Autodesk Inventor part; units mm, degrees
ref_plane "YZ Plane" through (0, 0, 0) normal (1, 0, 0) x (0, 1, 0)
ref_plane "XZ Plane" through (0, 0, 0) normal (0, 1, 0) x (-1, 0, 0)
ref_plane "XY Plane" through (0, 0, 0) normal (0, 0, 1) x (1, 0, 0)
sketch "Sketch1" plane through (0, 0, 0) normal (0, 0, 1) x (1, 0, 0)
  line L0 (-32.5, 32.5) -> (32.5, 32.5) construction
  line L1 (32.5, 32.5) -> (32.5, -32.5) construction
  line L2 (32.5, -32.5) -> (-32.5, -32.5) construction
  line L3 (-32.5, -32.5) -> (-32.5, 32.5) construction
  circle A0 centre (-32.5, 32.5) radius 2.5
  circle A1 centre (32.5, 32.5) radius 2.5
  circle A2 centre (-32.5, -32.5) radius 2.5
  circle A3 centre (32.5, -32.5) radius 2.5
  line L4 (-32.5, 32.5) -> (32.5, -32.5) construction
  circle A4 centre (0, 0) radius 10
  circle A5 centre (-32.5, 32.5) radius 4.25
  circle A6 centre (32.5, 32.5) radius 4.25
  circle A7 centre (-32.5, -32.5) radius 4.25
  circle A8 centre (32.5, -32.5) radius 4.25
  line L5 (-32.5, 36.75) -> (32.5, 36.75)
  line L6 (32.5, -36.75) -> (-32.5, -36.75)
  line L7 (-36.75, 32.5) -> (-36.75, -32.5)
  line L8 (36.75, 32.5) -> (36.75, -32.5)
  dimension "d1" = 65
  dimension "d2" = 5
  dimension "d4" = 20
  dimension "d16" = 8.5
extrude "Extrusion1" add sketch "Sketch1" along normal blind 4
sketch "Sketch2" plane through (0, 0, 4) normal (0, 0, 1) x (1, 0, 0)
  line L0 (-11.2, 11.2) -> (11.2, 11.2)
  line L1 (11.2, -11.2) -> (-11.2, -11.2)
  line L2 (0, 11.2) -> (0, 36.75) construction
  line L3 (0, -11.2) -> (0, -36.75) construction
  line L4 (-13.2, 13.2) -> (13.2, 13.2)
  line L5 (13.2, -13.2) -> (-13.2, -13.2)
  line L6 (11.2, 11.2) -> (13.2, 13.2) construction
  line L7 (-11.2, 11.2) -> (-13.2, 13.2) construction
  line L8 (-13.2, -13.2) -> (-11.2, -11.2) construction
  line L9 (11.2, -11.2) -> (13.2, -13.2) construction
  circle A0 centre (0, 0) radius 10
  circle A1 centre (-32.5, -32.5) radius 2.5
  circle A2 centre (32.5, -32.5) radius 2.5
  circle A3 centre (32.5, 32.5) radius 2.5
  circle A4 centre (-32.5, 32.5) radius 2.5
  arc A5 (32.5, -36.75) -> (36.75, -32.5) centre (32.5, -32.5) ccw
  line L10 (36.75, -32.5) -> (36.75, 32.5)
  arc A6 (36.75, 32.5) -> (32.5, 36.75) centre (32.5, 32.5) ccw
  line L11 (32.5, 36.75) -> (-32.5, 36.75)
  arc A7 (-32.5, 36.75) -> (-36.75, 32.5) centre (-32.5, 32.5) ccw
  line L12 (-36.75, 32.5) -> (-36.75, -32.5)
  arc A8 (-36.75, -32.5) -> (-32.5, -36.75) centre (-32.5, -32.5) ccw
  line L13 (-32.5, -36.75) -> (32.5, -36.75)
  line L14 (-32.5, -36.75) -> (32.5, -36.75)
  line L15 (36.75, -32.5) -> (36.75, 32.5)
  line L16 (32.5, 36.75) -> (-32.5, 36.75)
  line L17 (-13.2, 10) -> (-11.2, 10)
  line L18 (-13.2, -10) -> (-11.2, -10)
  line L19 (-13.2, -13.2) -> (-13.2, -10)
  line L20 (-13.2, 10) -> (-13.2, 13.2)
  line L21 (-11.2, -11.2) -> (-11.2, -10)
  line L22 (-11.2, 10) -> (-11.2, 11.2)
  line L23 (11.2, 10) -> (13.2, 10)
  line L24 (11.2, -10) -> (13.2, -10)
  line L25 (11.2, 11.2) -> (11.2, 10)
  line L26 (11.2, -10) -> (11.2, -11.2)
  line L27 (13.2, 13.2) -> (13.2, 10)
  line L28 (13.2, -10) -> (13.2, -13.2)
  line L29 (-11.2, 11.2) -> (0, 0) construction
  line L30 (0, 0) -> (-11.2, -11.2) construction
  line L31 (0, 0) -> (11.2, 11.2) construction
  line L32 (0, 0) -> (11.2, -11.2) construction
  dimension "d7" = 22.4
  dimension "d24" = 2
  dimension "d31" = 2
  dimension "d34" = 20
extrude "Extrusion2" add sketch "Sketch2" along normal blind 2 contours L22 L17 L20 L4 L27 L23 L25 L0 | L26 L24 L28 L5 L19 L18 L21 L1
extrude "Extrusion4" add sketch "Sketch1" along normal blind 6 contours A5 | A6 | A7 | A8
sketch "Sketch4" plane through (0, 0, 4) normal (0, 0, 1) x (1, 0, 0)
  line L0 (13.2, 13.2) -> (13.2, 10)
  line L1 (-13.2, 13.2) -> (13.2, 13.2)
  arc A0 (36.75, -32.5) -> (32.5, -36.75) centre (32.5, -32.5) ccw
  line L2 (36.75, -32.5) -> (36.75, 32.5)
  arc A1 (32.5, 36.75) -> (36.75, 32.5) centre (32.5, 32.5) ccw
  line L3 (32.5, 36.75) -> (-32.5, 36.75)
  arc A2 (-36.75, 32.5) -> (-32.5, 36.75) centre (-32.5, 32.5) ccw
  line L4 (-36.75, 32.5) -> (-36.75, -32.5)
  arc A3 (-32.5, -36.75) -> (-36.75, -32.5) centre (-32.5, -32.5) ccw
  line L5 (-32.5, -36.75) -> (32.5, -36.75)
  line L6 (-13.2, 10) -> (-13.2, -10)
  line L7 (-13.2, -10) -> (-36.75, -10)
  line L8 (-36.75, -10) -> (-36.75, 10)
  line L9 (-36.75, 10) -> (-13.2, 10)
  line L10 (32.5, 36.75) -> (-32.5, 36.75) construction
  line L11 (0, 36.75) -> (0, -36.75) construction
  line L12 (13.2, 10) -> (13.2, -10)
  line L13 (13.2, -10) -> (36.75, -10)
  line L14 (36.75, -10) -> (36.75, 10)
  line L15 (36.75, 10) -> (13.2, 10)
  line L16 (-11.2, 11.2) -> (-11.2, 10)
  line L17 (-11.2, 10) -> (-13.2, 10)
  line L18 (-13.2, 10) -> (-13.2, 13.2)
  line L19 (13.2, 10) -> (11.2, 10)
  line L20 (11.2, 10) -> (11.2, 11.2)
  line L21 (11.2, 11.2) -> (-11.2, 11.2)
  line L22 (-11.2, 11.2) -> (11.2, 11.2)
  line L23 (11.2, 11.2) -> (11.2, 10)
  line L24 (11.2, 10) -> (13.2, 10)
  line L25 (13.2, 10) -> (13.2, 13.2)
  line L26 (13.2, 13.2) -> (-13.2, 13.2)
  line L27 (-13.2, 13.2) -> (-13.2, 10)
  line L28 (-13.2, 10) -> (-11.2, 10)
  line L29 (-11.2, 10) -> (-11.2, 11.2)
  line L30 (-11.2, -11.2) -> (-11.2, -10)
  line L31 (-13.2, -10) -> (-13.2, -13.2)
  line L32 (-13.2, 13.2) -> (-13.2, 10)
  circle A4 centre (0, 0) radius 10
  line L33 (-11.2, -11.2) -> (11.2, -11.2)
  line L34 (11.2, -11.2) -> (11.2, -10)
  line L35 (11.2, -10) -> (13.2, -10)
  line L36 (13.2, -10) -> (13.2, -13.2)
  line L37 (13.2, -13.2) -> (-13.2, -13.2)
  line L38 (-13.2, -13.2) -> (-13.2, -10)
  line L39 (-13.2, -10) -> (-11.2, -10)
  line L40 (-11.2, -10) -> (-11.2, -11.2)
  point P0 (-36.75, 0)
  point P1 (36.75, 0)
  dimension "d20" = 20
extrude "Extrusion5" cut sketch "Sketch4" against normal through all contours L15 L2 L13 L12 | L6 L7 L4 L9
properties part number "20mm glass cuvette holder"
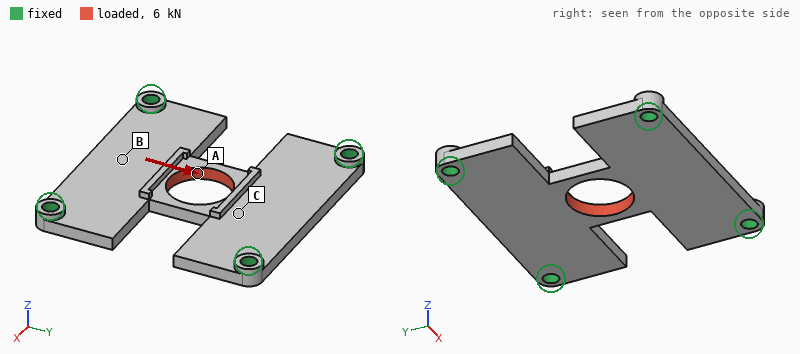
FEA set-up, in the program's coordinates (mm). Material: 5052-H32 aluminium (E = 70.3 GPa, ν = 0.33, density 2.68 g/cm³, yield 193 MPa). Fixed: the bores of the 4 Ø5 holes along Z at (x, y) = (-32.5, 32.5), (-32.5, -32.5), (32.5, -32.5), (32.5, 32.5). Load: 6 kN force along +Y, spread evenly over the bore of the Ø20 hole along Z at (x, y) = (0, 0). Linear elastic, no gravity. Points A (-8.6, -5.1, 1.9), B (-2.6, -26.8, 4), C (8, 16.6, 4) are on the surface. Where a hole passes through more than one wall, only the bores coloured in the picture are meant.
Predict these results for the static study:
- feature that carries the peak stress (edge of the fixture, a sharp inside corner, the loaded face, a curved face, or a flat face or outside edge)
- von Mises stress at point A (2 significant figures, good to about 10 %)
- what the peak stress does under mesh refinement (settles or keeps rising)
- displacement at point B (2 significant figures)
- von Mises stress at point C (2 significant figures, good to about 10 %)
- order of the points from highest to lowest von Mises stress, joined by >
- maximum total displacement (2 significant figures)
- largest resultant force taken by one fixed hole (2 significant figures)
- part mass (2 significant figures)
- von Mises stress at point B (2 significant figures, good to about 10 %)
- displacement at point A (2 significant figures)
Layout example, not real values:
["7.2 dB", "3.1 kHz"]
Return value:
["edge of the fixture", "42 MPa", "keeps rising", "27 µm", "26 MPa", "A > C > B", "30 µm", "1.9 kN", "45 g", "9.4 MPa", "28 µm"]
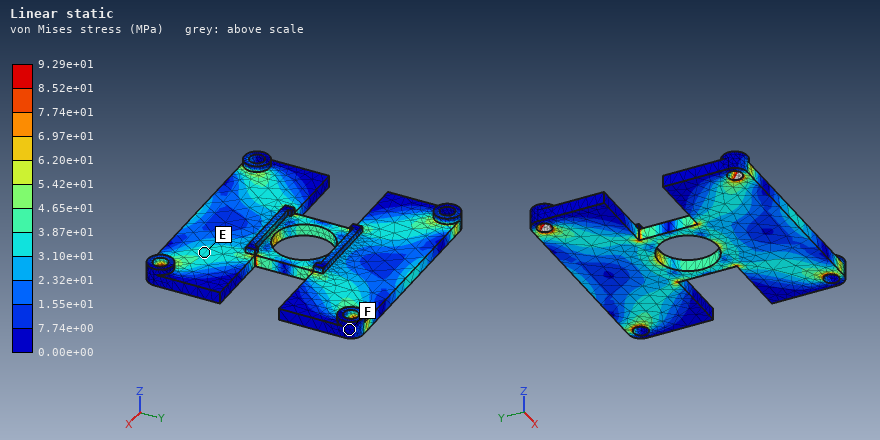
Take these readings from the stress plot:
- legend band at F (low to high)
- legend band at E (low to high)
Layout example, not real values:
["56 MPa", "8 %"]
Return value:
["0.00e+00 to 7.74e+00 MPa", "3.10e+01 to 3.87e+01 MPa"]
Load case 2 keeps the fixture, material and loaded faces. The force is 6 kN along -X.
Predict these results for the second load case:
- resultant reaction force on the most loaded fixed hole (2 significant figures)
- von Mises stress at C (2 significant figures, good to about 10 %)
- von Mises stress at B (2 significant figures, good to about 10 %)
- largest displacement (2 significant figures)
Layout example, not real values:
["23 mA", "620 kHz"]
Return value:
["1.8 kN", "21 MPa", "11 MPa", "42 µm"]
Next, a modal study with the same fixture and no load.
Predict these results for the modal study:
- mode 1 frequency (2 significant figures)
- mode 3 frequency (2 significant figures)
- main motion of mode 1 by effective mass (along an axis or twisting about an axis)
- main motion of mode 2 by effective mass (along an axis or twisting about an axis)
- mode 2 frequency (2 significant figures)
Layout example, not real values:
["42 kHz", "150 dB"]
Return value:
["3400 Hz", "6900 Hz", "along Z", "twisting about X", "5400 Hz"]
